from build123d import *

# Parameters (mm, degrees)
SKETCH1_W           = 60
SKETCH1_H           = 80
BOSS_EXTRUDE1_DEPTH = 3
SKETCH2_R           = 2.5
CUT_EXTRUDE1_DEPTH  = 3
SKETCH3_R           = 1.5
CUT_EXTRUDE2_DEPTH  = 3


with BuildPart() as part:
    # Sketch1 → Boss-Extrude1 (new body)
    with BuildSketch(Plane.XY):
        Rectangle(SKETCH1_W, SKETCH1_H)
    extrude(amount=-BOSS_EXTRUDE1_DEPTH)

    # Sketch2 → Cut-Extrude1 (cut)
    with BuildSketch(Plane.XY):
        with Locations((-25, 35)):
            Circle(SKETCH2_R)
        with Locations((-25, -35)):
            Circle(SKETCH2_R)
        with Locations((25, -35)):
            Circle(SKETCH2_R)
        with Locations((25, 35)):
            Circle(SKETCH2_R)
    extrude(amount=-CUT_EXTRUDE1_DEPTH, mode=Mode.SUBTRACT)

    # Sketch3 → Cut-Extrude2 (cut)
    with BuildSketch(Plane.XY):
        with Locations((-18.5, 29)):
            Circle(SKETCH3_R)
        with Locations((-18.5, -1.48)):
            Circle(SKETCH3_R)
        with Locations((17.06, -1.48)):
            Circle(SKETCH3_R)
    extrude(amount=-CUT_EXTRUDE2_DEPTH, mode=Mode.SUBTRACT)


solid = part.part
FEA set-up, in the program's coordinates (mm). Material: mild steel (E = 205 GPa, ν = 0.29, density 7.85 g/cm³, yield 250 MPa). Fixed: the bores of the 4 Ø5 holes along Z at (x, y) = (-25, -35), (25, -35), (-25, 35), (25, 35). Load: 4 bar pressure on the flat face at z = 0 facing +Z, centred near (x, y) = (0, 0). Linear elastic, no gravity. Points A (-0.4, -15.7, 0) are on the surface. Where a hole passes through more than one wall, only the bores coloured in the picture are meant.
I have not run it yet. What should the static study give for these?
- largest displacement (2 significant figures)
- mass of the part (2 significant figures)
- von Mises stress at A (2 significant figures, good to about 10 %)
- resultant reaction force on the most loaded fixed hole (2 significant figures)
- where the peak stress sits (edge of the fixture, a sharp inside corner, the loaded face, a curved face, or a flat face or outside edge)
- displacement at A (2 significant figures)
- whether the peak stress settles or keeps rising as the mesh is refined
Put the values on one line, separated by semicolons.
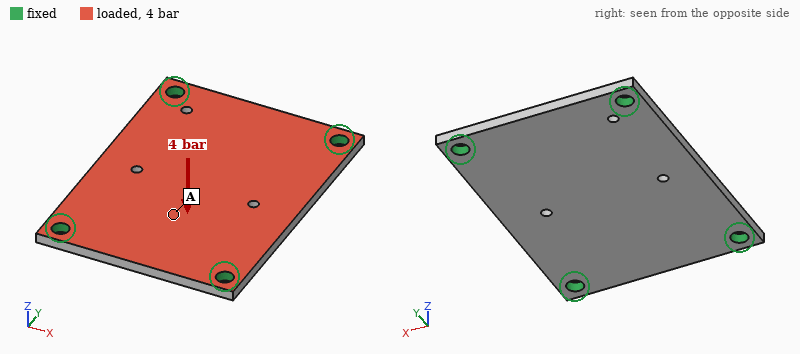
80 µm; 110 g; 37 MPa; 470 N; edge of the fixture; 62 µm; keeps rising
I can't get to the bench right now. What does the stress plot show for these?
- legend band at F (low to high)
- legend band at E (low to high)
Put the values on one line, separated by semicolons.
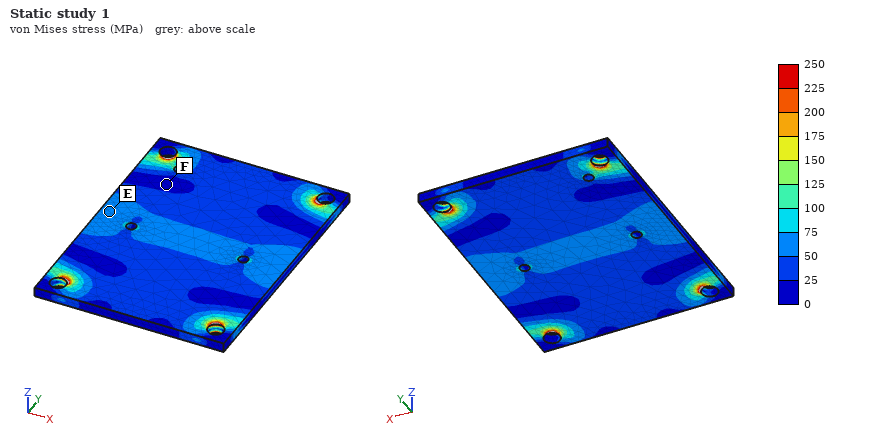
0 to 25 MPa; 50 to 75 MPa
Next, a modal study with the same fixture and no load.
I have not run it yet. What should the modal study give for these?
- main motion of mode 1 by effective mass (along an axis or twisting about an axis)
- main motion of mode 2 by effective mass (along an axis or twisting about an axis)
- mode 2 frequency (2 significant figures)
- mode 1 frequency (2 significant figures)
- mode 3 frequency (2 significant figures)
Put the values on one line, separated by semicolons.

along Z; twisting about Y; 4200 Hz; 2700 Hz; 6200 Hz
